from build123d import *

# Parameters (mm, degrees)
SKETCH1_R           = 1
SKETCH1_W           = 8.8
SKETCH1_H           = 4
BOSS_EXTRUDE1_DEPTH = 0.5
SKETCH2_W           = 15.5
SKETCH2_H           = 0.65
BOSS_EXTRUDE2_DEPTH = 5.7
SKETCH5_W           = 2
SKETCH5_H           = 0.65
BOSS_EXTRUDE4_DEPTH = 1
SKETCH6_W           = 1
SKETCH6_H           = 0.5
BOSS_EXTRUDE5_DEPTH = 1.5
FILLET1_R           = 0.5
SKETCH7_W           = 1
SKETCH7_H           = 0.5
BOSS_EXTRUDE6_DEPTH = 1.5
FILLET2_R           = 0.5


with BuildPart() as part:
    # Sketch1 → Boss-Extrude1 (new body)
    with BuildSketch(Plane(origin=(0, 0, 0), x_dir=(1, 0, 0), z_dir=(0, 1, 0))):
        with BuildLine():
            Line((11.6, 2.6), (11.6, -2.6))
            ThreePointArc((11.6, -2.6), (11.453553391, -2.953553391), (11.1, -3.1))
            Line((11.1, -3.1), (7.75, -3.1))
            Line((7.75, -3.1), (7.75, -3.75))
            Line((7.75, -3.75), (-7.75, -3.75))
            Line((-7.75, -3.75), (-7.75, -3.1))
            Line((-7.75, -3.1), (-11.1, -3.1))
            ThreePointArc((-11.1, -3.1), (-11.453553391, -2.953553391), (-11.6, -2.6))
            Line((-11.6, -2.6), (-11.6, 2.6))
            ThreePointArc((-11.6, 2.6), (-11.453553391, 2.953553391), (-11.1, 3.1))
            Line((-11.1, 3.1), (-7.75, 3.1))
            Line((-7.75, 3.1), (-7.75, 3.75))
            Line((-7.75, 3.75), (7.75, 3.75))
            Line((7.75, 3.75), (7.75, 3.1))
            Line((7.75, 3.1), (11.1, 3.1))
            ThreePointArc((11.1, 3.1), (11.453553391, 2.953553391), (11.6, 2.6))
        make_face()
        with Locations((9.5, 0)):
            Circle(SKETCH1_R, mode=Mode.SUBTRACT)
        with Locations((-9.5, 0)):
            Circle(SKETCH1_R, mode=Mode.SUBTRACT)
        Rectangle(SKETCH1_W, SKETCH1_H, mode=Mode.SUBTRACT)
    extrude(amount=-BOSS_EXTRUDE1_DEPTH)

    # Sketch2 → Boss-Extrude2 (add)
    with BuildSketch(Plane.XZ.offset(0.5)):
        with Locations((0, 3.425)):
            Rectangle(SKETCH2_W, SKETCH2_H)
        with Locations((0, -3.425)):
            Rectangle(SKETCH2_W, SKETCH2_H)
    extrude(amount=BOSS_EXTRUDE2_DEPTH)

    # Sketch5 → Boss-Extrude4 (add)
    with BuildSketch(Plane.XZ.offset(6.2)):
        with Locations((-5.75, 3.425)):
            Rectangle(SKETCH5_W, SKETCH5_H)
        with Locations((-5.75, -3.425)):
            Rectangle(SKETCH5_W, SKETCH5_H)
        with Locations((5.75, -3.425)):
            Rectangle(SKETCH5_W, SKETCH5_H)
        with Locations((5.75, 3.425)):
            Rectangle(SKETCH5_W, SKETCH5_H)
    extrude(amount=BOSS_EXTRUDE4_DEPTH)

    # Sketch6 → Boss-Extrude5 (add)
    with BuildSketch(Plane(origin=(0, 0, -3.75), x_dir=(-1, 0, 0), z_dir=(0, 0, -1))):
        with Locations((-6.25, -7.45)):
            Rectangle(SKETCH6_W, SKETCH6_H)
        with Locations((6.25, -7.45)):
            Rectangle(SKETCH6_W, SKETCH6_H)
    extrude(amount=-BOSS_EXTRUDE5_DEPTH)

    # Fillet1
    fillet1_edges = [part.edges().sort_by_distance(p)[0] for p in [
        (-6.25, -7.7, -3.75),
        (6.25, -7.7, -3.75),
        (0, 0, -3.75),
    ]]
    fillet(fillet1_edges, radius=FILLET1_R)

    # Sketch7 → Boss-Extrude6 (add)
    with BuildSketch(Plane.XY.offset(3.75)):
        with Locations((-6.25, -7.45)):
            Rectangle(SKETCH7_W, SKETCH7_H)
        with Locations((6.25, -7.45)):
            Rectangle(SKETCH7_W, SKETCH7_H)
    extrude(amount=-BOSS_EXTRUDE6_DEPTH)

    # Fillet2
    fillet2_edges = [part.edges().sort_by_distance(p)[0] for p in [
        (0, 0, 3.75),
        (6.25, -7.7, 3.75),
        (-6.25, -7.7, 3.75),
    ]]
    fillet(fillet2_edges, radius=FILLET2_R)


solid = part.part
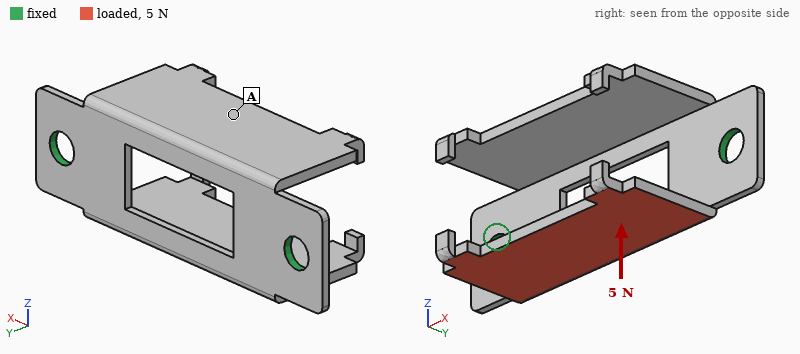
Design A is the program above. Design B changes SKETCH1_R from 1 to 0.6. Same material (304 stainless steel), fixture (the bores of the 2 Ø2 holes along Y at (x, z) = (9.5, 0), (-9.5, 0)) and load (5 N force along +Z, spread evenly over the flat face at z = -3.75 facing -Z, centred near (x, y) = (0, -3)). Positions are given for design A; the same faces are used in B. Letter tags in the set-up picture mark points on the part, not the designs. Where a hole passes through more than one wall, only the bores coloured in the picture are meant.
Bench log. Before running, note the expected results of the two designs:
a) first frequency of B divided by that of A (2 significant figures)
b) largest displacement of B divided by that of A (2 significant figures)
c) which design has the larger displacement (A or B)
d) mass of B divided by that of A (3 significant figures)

0.90
1.1
B
1.01
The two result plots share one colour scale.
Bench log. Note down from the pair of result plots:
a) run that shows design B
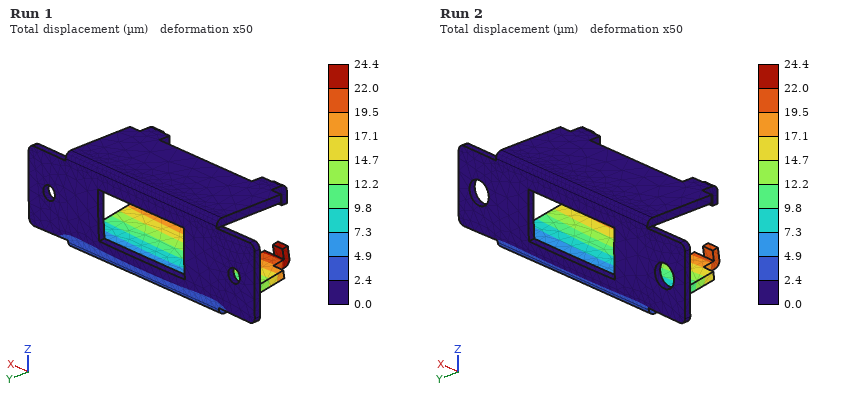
Run 1
